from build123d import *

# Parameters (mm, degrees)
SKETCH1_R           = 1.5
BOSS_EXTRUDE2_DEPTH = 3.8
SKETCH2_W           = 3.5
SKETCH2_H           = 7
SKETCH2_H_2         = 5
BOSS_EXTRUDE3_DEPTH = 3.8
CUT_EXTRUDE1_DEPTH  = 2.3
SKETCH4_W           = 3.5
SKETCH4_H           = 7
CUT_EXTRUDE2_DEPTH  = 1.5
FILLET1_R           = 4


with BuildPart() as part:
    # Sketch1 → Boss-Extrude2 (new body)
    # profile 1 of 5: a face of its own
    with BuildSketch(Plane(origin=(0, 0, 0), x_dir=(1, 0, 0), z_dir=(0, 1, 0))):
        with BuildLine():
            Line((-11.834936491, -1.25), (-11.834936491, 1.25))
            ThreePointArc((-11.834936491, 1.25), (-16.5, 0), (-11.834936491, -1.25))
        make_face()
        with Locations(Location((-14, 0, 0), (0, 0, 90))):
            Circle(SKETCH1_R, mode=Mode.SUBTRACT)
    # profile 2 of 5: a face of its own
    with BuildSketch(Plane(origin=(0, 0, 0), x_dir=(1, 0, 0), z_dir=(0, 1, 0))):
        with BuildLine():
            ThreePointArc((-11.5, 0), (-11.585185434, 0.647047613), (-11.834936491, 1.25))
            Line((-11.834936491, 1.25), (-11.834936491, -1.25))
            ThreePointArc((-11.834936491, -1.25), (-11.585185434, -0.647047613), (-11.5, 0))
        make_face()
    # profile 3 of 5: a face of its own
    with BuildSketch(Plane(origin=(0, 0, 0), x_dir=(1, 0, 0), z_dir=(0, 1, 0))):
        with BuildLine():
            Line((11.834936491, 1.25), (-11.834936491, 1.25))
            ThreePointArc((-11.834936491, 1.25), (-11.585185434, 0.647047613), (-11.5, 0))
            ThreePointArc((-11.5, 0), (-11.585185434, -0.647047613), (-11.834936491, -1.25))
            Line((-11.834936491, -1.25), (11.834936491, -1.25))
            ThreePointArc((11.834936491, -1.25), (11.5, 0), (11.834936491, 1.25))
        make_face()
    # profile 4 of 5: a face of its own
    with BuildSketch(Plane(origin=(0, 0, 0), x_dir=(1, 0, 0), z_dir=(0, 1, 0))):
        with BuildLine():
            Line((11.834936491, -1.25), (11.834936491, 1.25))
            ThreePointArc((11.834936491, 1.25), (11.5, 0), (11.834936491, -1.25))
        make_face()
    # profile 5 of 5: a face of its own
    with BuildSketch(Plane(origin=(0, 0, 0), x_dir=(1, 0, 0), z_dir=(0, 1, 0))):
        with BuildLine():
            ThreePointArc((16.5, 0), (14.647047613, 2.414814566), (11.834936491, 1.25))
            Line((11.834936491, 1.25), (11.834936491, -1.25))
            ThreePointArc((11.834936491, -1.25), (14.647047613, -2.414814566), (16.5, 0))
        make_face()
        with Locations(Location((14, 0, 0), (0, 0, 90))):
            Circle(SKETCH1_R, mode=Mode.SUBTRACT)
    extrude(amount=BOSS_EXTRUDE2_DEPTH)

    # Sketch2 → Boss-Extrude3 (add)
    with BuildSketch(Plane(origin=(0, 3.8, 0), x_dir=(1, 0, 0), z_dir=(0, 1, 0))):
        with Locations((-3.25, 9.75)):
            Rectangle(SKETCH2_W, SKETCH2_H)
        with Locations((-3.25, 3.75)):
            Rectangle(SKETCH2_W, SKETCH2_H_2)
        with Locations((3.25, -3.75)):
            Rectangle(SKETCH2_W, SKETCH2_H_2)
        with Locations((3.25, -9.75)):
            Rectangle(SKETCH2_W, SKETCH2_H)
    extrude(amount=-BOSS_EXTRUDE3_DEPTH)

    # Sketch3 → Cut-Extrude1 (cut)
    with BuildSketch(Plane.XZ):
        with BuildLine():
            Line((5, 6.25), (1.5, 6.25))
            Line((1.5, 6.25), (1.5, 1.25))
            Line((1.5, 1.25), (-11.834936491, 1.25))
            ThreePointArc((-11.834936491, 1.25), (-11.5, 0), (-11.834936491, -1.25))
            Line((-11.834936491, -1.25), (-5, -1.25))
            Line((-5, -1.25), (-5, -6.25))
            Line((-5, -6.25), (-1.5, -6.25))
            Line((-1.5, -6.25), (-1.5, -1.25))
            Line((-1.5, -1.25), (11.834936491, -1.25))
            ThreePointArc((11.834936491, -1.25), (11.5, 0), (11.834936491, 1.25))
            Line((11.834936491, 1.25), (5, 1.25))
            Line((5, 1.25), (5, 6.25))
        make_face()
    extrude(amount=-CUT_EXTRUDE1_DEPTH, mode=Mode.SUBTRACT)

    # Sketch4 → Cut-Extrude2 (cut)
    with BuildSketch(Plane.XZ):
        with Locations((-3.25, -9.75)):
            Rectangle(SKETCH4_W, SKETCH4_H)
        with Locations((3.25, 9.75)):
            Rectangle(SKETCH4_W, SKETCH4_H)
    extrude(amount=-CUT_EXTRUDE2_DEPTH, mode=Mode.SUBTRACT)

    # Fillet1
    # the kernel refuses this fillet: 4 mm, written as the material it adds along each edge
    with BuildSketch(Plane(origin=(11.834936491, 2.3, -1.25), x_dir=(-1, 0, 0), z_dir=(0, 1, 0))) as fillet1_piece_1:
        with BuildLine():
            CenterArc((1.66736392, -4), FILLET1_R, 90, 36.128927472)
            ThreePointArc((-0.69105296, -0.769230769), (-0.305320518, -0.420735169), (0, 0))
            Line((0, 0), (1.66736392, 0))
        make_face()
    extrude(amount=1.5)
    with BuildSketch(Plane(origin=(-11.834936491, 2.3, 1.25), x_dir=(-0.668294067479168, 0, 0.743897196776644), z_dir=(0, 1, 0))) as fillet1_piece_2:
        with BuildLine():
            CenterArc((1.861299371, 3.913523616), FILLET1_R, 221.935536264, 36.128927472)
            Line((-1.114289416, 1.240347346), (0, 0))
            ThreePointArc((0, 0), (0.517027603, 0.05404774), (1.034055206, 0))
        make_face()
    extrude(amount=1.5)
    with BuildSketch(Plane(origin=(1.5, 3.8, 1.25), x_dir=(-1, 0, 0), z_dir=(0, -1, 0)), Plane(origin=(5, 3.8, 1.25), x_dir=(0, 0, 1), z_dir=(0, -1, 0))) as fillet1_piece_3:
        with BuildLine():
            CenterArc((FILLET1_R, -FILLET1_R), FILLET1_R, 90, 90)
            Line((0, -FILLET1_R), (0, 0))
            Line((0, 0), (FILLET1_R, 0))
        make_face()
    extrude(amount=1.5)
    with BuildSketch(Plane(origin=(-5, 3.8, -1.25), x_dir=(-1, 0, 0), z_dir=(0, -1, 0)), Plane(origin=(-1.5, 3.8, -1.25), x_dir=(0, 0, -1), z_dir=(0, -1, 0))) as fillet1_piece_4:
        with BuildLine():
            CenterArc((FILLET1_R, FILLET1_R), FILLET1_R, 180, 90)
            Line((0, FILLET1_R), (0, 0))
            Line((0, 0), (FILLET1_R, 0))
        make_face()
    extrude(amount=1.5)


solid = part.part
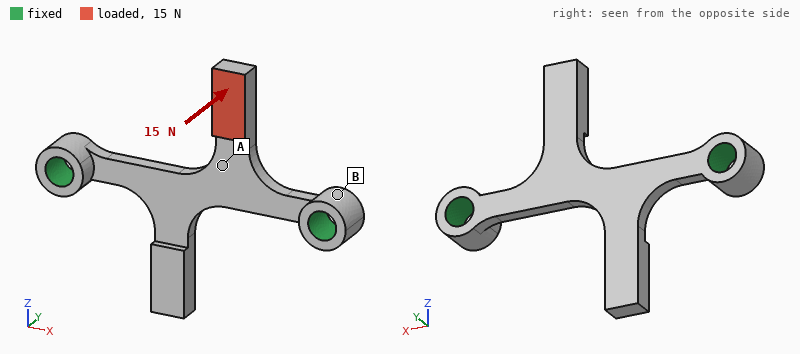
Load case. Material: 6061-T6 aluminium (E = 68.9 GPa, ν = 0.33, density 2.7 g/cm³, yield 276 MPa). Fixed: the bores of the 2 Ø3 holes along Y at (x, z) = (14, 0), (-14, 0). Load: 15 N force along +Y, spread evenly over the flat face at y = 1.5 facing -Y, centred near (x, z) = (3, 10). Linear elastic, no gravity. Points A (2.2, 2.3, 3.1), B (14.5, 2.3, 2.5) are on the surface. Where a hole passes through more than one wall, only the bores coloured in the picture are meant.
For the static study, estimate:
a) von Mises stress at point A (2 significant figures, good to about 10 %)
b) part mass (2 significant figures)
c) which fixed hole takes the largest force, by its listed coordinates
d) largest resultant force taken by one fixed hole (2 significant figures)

66 MPa
1.00 g
(14, 0)
11 N
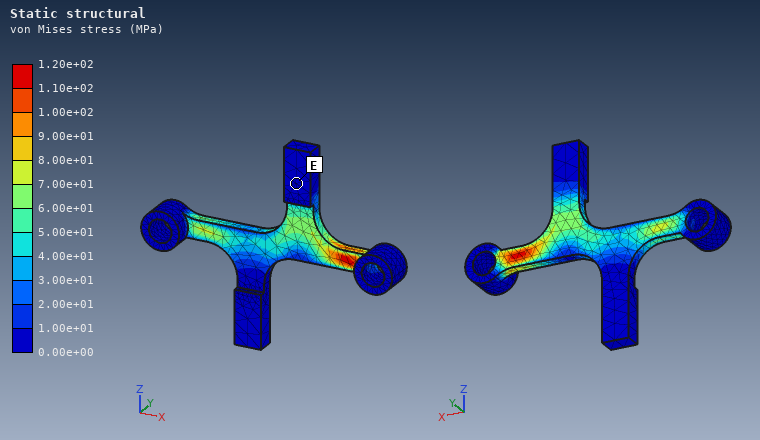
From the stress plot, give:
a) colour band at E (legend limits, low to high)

0.00e+00 to 1.00e+01 MPa
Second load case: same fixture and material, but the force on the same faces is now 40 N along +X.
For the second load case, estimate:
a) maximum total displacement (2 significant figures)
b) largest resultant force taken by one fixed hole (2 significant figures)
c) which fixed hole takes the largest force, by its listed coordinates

51 µm
39 N
(14, 0)
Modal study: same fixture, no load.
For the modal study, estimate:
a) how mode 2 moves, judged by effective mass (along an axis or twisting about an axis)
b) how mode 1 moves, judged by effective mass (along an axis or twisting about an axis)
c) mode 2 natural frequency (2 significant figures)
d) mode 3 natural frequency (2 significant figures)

along Y
twisting about X
4600 Hz
11 kHz
